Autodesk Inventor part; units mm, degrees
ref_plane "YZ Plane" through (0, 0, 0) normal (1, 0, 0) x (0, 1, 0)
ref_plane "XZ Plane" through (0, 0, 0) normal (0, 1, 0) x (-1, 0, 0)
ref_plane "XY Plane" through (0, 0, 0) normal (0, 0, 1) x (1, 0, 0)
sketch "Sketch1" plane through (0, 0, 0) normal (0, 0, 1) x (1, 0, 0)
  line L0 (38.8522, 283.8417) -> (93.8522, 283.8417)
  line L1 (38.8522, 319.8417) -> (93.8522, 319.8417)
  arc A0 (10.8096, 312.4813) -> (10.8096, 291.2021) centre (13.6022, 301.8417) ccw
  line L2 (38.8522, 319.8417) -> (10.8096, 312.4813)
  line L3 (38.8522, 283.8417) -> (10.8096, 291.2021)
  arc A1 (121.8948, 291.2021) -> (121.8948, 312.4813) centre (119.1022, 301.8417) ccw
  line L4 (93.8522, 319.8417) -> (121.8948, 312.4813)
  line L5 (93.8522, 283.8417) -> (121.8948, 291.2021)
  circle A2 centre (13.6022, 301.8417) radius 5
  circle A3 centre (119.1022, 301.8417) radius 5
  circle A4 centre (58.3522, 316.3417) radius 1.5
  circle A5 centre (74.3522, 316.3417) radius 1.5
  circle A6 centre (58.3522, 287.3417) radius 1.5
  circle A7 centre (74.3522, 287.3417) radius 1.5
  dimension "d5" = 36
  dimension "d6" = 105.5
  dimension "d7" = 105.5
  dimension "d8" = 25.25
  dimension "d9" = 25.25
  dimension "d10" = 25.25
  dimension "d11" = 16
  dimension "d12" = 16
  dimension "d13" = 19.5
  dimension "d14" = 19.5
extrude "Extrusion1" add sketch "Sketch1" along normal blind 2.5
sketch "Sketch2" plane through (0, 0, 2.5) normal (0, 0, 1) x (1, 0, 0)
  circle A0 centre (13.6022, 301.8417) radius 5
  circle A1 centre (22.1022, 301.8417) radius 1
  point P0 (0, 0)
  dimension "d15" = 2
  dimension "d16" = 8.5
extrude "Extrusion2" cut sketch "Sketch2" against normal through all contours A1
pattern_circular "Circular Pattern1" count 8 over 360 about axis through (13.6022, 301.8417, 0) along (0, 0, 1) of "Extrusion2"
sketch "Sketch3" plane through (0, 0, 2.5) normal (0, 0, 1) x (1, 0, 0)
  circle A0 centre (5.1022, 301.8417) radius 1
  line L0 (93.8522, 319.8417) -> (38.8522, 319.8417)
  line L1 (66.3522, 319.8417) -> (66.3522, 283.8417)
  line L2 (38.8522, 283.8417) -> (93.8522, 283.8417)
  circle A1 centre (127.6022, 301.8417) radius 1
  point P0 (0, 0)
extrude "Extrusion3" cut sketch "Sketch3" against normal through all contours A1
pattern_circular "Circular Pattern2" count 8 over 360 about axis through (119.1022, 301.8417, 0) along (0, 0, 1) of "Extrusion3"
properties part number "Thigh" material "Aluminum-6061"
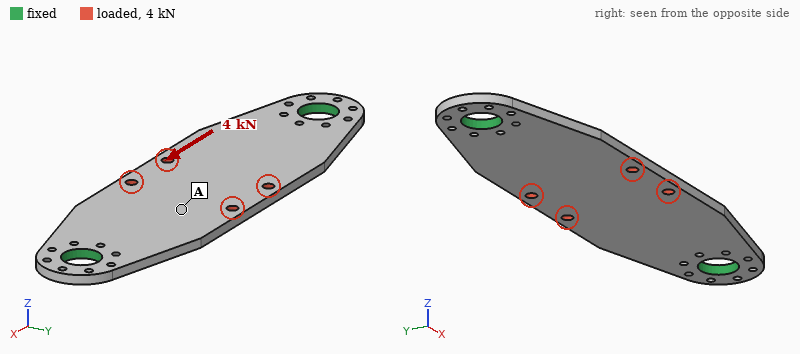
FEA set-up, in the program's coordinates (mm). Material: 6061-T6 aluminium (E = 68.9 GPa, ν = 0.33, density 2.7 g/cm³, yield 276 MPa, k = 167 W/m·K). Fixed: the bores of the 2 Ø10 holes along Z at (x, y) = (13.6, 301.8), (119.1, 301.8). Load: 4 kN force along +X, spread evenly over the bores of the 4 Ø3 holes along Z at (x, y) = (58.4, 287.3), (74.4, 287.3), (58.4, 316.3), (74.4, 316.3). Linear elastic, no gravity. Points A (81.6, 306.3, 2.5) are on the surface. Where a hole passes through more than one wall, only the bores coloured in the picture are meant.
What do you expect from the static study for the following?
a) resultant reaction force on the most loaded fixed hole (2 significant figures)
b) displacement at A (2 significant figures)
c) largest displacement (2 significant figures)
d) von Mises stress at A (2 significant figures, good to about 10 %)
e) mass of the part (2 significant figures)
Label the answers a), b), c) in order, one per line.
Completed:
a) 2.0 kN
b) 15 µm
c) 22 µm
d) 16 MPa
e) 24 g
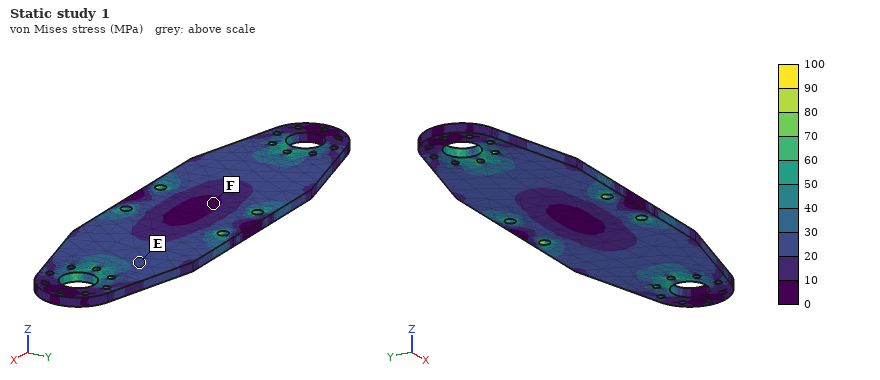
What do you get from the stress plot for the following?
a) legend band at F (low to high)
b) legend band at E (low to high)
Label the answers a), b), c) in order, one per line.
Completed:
a) 0 to 10 MPa
b) 20 to 30 MPa
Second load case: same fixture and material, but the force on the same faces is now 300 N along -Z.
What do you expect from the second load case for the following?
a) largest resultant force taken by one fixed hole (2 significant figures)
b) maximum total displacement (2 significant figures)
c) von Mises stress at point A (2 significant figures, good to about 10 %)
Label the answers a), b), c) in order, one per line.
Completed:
a) 150 N
b) 0.57 mm
c) 51 MPa
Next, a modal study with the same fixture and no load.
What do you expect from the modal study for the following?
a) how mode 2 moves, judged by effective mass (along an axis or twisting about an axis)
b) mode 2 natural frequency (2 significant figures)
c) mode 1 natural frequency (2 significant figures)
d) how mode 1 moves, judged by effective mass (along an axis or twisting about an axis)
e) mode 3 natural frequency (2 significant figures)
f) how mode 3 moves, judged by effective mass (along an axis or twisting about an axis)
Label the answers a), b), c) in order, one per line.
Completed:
a) twisting about X
b) 2100 Hz
c) 1200 Hz
d) along Z
e) 3300 Hz
f) twisting about Y
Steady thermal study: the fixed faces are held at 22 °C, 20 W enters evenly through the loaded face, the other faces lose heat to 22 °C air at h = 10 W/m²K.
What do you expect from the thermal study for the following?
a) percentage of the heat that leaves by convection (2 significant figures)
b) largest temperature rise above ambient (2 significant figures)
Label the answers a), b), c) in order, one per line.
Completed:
a) 7.3 %
b) 35 K
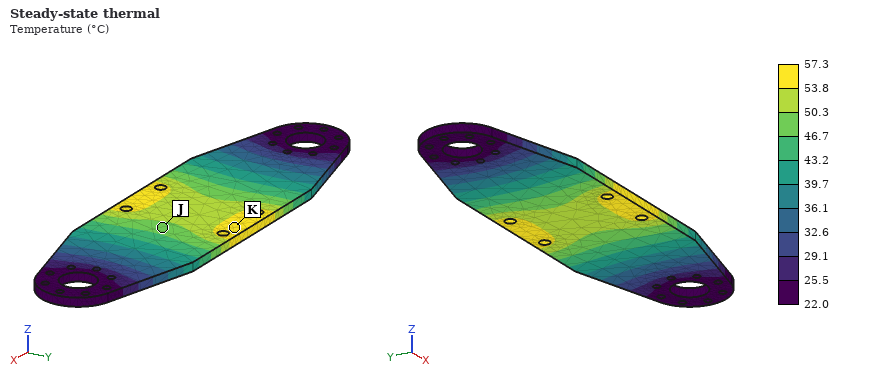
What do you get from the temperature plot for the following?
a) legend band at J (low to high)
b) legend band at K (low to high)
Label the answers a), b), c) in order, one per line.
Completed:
a) 46.7 to 50.3 °C
b) 53.8 to 57.3 °C
